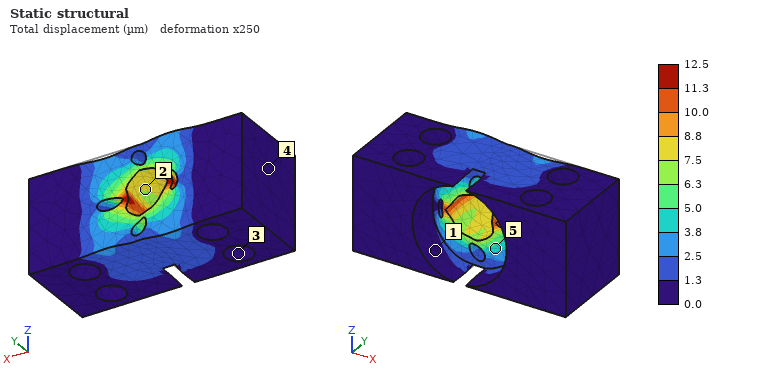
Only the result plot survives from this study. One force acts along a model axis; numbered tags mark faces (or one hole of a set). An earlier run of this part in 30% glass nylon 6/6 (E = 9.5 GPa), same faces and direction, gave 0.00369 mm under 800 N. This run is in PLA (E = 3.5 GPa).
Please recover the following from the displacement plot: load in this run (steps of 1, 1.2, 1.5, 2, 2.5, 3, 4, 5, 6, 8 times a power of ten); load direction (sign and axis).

1 kN
-X
